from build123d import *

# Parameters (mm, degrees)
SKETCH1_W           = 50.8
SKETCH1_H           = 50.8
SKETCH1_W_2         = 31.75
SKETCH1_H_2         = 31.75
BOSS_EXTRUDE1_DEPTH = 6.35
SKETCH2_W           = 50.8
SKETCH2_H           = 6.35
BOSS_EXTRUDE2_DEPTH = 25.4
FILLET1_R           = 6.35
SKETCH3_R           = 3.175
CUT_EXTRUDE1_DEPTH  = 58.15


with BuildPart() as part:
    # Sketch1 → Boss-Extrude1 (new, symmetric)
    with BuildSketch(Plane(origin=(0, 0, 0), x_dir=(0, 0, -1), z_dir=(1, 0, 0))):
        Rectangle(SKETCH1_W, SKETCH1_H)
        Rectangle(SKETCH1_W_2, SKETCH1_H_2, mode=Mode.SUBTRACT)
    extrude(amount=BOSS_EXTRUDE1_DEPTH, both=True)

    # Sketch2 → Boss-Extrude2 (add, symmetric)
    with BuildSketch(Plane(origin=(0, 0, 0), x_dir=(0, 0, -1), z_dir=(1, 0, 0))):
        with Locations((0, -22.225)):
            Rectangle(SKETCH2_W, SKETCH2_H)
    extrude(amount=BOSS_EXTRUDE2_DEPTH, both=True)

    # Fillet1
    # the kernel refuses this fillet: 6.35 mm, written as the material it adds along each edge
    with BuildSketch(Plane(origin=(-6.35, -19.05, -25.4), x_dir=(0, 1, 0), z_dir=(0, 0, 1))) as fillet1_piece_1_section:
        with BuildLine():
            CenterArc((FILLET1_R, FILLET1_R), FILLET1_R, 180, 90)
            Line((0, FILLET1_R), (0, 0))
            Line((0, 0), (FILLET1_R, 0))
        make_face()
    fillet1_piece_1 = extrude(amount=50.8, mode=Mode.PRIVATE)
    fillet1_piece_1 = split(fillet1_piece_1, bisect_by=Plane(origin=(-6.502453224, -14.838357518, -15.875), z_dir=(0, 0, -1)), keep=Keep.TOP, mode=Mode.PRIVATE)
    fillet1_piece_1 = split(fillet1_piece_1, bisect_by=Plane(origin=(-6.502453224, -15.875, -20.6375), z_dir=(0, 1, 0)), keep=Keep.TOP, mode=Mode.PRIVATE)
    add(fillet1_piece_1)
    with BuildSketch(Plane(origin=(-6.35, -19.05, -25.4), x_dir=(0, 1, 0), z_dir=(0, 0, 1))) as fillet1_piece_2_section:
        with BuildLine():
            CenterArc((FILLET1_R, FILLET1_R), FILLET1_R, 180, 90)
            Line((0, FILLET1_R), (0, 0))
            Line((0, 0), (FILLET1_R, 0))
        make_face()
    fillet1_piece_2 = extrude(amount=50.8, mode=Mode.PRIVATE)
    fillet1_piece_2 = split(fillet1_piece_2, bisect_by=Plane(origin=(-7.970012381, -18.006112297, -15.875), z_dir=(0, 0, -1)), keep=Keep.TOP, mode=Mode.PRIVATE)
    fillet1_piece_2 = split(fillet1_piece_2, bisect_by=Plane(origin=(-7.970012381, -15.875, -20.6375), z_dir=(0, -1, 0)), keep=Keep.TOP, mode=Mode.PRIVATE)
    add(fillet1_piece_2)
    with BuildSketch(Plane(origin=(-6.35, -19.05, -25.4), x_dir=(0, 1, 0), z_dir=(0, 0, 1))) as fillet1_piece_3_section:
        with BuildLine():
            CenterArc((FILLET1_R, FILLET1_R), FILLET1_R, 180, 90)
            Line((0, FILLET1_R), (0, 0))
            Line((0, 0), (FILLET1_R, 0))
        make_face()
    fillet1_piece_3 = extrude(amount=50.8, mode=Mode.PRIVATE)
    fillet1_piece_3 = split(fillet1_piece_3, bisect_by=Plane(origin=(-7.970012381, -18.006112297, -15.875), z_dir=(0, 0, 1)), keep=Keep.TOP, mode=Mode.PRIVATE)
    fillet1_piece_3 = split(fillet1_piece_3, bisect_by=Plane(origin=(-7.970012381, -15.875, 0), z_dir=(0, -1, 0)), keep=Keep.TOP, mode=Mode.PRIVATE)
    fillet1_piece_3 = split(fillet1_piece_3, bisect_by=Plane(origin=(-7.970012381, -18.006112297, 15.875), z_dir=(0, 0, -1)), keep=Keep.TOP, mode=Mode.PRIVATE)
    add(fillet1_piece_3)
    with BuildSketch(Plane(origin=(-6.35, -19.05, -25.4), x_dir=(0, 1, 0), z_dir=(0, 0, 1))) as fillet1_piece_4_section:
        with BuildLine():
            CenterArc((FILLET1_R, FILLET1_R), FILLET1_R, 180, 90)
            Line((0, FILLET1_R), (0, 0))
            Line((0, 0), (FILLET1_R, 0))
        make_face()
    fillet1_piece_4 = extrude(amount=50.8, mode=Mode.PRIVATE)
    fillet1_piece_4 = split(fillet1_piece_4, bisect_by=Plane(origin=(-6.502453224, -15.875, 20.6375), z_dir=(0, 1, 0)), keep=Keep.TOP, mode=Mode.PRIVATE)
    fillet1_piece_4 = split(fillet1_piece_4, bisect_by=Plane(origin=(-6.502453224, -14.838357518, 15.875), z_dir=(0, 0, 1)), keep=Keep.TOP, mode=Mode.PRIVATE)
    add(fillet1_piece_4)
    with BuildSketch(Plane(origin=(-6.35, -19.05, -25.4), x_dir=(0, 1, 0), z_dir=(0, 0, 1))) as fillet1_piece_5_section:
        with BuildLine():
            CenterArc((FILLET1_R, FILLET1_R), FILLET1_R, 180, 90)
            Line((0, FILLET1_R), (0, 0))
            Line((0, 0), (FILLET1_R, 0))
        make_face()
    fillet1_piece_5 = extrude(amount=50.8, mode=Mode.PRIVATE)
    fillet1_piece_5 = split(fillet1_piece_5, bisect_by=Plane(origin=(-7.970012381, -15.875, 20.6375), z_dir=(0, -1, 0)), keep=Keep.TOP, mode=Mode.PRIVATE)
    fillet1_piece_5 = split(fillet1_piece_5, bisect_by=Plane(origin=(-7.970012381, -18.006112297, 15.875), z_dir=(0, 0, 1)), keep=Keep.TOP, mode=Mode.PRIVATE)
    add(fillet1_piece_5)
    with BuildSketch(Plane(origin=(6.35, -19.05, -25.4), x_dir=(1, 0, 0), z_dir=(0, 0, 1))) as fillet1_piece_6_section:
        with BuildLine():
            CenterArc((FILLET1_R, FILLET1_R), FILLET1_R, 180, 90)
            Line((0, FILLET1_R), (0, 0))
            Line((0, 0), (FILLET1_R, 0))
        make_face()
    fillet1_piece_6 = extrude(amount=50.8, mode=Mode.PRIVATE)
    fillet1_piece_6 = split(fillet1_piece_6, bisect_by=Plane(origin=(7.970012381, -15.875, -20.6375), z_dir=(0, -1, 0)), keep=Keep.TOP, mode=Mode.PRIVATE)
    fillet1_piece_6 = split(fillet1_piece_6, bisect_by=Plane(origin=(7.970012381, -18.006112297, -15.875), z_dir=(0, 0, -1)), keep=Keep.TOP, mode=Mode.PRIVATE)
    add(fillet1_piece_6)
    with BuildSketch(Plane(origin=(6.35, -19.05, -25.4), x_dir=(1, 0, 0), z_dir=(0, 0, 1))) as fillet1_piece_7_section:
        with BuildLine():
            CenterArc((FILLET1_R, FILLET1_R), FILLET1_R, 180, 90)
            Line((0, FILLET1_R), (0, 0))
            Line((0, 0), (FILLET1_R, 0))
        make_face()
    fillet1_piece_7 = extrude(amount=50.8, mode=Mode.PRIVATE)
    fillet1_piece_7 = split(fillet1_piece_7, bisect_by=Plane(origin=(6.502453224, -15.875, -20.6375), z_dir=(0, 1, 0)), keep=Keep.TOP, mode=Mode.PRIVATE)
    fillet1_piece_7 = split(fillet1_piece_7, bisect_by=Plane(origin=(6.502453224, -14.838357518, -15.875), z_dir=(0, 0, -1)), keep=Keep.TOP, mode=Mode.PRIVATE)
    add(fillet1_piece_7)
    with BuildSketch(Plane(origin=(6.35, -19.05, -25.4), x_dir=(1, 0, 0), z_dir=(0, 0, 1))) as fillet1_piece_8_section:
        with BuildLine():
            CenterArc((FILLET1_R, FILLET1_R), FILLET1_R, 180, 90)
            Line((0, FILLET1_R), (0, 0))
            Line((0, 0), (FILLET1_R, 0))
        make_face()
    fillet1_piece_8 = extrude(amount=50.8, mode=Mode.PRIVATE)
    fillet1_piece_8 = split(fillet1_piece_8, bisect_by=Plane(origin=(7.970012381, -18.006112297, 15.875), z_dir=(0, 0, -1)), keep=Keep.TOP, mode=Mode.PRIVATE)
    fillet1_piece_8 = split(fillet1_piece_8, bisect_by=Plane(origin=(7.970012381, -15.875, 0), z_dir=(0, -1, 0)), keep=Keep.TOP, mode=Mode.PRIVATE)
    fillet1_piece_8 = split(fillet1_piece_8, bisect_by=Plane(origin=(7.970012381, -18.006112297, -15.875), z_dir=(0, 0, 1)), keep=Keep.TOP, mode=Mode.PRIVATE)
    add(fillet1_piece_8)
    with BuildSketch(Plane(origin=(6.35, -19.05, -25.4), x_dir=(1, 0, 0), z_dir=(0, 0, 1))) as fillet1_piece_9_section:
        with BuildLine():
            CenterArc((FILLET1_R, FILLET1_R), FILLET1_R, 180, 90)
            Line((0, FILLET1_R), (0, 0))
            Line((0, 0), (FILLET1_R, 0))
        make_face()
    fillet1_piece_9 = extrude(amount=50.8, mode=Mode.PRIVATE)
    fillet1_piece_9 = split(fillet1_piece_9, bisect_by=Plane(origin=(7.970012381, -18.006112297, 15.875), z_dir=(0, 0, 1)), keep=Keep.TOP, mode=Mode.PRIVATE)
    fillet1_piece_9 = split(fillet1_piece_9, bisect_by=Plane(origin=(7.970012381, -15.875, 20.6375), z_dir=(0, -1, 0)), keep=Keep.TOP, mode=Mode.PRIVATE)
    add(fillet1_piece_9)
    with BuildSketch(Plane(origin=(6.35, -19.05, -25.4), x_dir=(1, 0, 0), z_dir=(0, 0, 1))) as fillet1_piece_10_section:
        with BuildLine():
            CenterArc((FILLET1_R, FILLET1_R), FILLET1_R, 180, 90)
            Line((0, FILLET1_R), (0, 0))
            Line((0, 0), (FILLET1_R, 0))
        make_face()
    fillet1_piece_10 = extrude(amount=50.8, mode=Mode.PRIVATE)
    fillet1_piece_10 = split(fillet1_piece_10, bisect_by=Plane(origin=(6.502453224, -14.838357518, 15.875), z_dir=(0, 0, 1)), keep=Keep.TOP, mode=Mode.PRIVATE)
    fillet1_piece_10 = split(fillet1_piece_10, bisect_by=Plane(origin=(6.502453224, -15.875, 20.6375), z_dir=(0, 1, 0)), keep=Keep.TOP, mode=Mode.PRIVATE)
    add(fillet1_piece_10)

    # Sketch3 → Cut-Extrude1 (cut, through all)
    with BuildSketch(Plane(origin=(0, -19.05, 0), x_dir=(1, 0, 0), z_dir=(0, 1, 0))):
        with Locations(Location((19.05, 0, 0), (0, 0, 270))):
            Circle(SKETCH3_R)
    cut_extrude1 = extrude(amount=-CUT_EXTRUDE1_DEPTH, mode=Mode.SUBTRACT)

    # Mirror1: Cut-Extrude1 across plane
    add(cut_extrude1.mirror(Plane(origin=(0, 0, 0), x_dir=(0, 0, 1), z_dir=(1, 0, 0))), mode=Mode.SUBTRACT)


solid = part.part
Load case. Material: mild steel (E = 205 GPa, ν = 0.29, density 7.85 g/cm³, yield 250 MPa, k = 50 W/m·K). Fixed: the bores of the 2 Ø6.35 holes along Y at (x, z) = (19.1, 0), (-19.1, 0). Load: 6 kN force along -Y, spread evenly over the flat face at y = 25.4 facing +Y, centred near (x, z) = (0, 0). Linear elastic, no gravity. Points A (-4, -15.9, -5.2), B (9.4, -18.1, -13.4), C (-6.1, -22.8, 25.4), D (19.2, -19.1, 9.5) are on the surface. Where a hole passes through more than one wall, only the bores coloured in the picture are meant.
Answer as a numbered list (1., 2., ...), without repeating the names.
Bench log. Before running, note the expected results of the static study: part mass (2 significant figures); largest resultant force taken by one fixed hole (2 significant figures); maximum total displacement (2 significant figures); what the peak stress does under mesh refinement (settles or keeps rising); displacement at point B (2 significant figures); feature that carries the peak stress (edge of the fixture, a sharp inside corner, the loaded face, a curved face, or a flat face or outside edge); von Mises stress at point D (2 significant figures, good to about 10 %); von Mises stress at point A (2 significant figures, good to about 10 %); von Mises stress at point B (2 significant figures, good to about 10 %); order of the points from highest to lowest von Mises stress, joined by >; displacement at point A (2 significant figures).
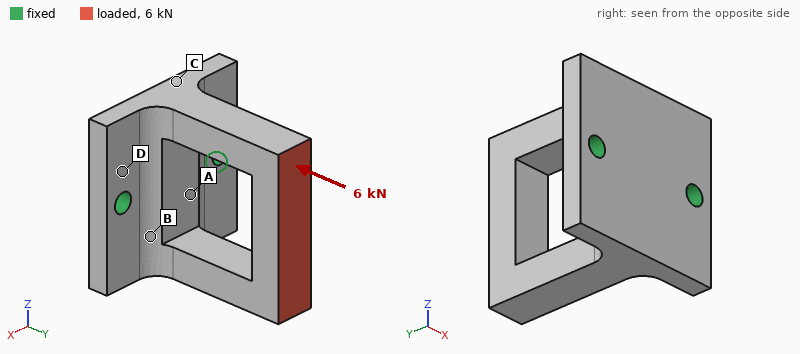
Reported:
1. 260 g
2. 3.3 kN
3. 41 µm
4. keeps rising
5. 13 µm
6. edge of the fixture
7. 39 MPa
8. 89 MPa
9. 57 MPa
10. A > B > D > C
11. 8.6 µm
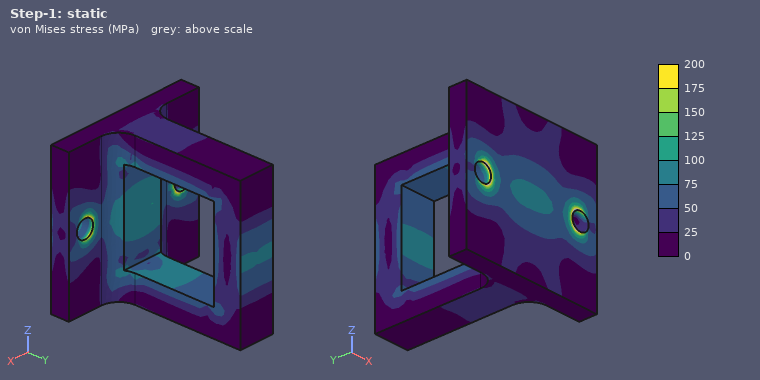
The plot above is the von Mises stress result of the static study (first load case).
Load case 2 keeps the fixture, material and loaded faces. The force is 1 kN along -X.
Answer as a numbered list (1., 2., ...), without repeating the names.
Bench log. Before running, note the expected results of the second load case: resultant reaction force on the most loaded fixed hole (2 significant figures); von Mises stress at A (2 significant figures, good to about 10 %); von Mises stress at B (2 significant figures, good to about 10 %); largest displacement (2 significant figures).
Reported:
1. 1.5 kN
2. 20 MPa
3. 52 MPa
4. 73 µm
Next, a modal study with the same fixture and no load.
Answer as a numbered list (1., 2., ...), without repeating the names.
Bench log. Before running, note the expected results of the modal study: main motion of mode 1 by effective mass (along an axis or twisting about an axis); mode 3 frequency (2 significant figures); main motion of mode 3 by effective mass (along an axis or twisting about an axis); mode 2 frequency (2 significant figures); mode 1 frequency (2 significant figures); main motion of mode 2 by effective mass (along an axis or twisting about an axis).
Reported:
1. along Z
2. 5500 Hz
3. twisting about Y
4. 2700 Hz
5. 2100 Hz
6. along X
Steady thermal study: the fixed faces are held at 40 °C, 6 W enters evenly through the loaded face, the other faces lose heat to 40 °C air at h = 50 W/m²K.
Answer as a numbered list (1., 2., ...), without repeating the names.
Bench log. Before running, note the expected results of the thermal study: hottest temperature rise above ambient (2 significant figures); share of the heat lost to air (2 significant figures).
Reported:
1. 18 K
2. 50 %
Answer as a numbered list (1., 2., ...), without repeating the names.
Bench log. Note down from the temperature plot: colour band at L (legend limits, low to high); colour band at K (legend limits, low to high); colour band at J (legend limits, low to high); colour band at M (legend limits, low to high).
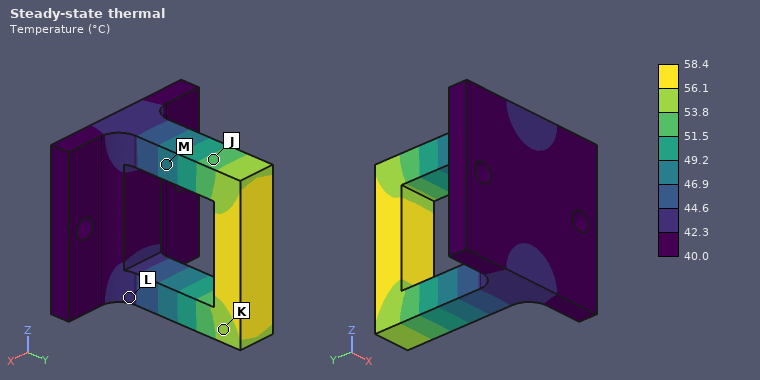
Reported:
1. 42.3 to 44.6 °C
2. 53.8 to 56.1 °C
3. 51.5 to 53.8 °C
4. 46.9 to 49.2 °C
